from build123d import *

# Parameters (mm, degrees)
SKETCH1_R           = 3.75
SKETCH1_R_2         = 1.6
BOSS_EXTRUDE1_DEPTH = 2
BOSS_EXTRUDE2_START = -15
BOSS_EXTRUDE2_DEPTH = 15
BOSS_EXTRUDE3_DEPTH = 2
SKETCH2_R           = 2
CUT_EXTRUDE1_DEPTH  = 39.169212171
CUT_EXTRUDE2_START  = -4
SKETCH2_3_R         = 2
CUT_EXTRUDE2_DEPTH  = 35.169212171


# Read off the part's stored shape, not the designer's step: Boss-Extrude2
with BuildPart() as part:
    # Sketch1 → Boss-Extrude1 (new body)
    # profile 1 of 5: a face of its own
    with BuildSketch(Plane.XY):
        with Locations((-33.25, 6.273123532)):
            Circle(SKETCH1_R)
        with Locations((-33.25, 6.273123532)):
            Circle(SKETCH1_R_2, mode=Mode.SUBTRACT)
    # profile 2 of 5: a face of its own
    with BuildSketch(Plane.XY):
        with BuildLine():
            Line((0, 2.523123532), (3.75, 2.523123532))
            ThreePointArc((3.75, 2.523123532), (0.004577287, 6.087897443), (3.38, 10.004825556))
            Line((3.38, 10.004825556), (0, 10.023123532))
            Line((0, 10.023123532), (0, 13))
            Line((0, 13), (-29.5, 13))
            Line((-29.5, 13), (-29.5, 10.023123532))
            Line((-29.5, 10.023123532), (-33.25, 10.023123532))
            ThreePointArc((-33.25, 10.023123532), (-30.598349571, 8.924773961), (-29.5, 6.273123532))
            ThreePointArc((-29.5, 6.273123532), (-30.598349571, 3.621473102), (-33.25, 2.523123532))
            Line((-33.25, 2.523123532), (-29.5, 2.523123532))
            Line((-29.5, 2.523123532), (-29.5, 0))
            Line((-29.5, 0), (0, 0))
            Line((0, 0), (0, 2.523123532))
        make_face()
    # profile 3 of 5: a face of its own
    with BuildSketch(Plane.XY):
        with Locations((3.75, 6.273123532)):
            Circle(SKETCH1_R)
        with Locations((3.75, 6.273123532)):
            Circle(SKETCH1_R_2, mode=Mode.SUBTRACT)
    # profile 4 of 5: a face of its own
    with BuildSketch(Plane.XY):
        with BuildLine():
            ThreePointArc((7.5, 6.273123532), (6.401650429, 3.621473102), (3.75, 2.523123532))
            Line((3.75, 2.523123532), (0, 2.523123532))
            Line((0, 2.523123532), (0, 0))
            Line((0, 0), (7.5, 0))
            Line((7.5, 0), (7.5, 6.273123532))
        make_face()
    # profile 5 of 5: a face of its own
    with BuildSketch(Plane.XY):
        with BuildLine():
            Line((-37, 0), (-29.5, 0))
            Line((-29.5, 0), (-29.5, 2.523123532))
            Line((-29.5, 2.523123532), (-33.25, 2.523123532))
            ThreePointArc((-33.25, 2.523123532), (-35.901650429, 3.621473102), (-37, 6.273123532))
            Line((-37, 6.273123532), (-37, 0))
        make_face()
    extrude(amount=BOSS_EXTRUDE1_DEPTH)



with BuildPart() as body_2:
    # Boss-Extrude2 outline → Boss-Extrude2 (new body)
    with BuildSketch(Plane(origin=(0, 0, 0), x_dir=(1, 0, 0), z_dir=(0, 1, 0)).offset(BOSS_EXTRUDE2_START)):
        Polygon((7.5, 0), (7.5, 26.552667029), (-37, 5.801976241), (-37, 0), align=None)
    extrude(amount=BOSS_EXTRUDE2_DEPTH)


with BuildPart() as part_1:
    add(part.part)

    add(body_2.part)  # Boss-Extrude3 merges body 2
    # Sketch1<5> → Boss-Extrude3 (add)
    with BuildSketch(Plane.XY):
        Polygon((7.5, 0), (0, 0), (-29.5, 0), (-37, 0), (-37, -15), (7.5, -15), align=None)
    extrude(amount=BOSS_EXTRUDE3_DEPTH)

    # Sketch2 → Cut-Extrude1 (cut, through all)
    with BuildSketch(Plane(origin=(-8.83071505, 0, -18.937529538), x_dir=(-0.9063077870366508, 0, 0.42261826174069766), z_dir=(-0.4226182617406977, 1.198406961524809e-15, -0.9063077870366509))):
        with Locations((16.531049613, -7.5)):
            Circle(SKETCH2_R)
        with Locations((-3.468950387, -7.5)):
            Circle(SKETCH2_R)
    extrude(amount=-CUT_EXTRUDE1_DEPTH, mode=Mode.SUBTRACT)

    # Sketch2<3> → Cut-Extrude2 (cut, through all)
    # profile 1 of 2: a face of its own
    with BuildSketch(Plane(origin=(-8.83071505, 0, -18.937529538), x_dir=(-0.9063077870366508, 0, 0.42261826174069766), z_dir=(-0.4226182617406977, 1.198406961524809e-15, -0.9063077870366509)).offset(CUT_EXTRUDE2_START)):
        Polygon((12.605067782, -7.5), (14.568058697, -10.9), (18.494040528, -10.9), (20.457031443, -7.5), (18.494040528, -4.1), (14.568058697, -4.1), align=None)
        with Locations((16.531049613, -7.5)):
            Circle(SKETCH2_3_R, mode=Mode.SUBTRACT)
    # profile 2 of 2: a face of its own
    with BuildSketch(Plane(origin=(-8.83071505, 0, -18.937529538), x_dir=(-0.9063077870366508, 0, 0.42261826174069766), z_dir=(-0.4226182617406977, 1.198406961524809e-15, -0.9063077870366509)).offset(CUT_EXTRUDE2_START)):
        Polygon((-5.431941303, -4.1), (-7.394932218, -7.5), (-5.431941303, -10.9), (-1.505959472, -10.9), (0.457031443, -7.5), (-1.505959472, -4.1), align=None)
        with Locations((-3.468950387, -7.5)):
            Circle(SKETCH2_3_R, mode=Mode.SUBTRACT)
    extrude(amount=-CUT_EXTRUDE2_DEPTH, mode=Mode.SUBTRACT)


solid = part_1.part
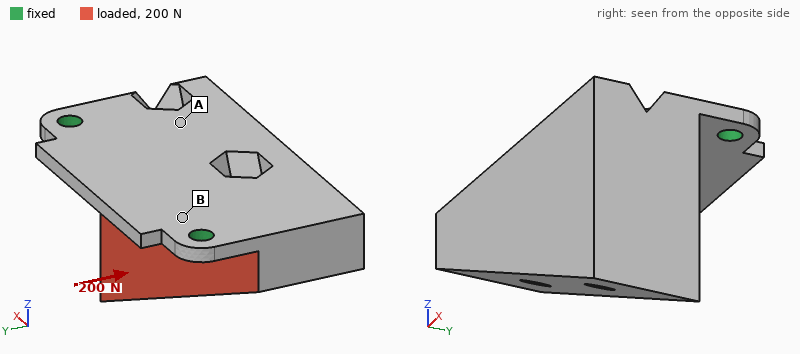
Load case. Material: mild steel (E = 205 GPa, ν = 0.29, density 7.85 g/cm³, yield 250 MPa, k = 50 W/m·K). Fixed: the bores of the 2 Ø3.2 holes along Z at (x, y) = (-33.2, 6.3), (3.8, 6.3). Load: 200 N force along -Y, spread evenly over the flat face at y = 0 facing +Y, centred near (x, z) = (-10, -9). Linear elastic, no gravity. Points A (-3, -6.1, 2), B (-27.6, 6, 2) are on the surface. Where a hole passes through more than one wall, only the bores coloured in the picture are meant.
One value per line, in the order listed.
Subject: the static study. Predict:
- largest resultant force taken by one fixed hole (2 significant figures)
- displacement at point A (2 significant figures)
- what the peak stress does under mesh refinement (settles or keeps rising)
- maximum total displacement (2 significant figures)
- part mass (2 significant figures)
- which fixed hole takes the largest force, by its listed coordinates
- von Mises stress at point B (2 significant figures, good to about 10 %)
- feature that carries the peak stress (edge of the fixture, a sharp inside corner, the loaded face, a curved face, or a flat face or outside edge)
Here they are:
130 N
0.028 mm
keeps rising
0.10 mm
92 g
(3.8, 6.3)
46 MPa
edge of the fixture
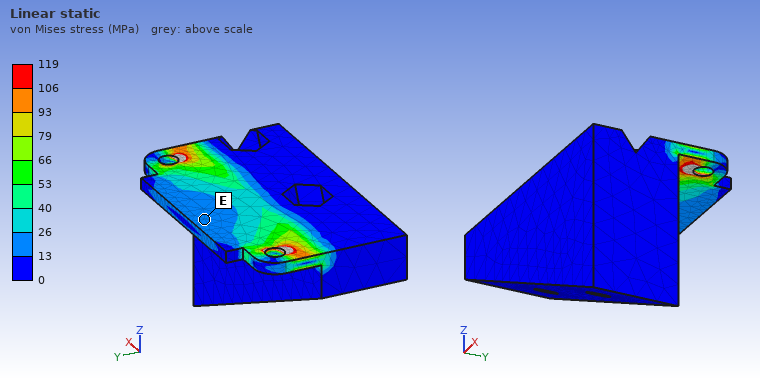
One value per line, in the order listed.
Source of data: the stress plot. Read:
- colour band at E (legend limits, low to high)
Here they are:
13 to 26 MPa
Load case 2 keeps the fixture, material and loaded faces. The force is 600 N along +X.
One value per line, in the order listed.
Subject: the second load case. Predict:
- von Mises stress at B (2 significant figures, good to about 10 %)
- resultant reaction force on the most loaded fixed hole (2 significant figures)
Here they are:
11 MPa
360 N
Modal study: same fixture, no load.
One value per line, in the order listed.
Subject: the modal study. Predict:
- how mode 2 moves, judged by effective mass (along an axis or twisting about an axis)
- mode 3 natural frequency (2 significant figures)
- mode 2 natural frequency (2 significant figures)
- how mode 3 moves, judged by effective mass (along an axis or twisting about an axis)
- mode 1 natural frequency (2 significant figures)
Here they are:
along X
6400 Hz
5000 Hz
along Z
870 Hz
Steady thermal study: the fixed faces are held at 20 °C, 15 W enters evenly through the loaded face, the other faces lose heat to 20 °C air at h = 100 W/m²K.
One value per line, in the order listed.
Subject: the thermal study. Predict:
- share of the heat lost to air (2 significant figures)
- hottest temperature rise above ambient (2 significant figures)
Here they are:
59 %
27 K
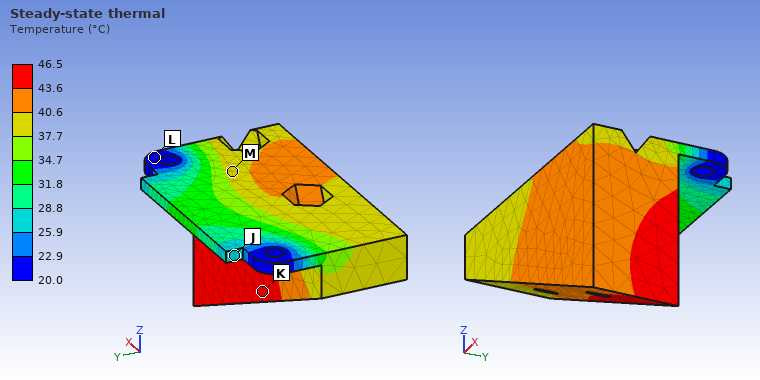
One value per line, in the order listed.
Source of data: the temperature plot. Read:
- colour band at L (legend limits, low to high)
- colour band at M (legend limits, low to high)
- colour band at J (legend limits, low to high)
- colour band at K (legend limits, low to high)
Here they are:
20.0 to 22.9 °C
37.7 to 40.6 °C
25.9 to 28.8 °C
43.6 to 46.5 °C
